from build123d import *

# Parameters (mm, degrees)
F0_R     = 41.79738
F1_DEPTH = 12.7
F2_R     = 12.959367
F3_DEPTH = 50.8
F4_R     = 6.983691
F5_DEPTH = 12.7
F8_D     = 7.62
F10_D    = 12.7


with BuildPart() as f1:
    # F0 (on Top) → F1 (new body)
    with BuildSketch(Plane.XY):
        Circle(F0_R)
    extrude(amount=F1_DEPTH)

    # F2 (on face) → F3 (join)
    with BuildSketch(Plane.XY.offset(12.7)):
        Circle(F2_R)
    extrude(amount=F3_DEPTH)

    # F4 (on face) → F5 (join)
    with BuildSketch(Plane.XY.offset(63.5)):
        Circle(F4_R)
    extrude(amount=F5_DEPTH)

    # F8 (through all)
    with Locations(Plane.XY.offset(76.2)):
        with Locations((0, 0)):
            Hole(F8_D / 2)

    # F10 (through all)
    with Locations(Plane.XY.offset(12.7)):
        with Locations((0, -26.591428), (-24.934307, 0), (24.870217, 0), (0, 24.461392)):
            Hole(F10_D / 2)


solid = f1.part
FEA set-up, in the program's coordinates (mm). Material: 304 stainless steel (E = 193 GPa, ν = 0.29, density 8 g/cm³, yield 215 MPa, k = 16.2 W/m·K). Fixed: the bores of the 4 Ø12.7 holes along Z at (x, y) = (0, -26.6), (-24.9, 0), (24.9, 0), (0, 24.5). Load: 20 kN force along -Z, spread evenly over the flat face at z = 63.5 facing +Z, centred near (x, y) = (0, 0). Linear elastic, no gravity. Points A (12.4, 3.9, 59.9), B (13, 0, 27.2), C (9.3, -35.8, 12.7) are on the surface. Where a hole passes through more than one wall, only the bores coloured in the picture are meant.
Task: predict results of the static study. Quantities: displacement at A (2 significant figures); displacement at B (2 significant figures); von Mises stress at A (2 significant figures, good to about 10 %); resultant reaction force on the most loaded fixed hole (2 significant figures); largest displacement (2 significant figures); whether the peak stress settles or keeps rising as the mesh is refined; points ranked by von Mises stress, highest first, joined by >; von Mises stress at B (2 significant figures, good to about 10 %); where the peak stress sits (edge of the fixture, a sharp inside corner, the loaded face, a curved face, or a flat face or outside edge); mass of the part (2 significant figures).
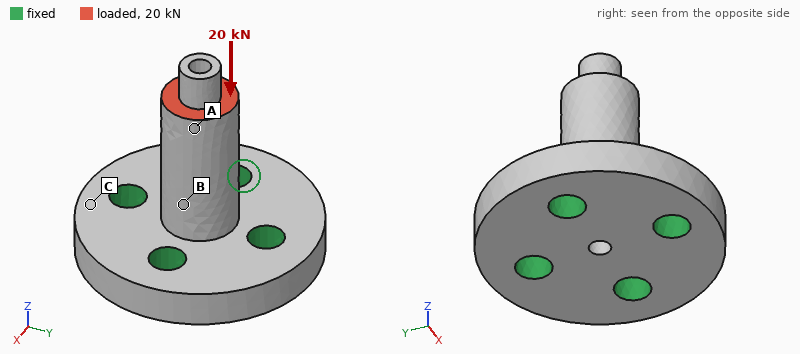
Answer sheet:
15 µm
7.4 µm
54 MPa
5.4 kN
16 µm
keeps rising
A > B > C
40 MPa
edge of the fixture
710 g
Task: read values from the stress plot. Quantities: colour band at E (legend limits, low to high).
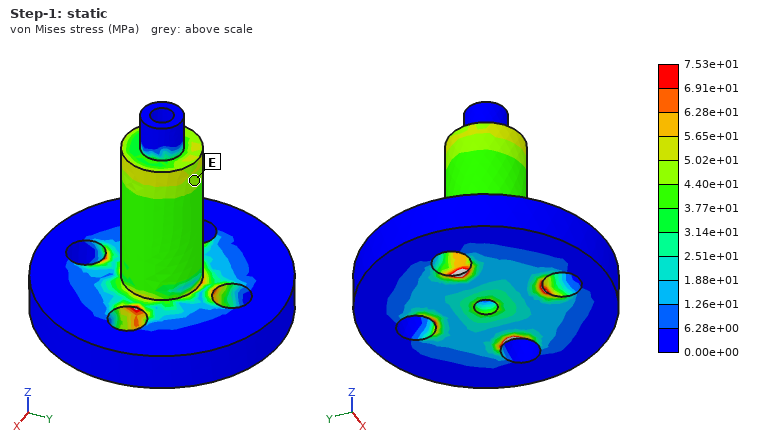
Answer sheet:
4.40e+01 to 5.02e+01 MPa
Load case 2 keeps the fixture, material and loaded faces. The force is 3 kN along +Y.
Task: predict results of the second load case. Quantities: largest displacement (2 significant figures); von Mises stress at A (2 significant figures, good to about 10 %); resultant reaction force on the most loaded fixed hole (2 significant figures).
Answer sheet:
67 µm
12 MPa
4.5 kN
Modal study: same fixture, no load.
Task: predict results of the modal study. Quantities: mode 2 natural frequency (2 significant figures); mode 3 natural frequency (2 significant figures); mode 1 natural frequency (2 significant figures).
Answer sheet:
4500 Hz
14 kHz
4500 Hz
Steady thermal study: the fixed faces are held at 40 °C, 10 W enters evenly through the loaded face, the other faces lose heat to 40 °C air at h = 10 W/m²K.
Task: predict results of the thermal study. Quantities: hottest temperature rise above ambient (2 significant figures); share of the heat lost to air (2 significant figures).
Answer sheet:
63 K
24 %
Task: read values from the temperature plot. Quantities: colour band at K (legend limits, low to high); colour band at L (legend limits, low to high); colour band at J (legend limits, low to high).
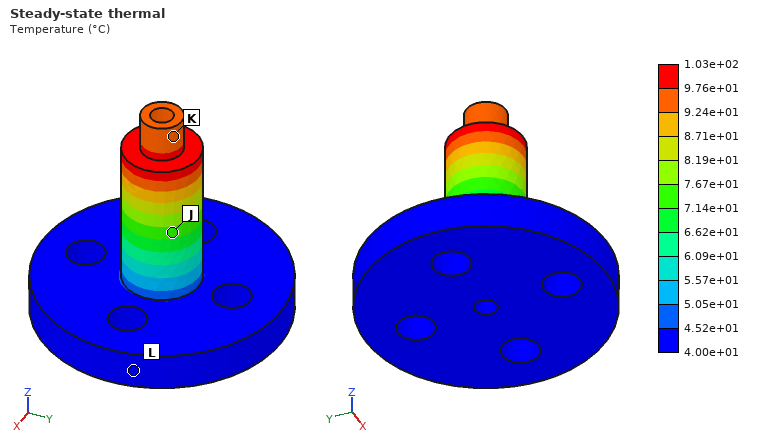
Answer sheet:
9.24e+01 to 9.76e+01 °C
4.00e+01 to 4.52e+01 °C
7.14e+01 to 7.67e+01 °C
